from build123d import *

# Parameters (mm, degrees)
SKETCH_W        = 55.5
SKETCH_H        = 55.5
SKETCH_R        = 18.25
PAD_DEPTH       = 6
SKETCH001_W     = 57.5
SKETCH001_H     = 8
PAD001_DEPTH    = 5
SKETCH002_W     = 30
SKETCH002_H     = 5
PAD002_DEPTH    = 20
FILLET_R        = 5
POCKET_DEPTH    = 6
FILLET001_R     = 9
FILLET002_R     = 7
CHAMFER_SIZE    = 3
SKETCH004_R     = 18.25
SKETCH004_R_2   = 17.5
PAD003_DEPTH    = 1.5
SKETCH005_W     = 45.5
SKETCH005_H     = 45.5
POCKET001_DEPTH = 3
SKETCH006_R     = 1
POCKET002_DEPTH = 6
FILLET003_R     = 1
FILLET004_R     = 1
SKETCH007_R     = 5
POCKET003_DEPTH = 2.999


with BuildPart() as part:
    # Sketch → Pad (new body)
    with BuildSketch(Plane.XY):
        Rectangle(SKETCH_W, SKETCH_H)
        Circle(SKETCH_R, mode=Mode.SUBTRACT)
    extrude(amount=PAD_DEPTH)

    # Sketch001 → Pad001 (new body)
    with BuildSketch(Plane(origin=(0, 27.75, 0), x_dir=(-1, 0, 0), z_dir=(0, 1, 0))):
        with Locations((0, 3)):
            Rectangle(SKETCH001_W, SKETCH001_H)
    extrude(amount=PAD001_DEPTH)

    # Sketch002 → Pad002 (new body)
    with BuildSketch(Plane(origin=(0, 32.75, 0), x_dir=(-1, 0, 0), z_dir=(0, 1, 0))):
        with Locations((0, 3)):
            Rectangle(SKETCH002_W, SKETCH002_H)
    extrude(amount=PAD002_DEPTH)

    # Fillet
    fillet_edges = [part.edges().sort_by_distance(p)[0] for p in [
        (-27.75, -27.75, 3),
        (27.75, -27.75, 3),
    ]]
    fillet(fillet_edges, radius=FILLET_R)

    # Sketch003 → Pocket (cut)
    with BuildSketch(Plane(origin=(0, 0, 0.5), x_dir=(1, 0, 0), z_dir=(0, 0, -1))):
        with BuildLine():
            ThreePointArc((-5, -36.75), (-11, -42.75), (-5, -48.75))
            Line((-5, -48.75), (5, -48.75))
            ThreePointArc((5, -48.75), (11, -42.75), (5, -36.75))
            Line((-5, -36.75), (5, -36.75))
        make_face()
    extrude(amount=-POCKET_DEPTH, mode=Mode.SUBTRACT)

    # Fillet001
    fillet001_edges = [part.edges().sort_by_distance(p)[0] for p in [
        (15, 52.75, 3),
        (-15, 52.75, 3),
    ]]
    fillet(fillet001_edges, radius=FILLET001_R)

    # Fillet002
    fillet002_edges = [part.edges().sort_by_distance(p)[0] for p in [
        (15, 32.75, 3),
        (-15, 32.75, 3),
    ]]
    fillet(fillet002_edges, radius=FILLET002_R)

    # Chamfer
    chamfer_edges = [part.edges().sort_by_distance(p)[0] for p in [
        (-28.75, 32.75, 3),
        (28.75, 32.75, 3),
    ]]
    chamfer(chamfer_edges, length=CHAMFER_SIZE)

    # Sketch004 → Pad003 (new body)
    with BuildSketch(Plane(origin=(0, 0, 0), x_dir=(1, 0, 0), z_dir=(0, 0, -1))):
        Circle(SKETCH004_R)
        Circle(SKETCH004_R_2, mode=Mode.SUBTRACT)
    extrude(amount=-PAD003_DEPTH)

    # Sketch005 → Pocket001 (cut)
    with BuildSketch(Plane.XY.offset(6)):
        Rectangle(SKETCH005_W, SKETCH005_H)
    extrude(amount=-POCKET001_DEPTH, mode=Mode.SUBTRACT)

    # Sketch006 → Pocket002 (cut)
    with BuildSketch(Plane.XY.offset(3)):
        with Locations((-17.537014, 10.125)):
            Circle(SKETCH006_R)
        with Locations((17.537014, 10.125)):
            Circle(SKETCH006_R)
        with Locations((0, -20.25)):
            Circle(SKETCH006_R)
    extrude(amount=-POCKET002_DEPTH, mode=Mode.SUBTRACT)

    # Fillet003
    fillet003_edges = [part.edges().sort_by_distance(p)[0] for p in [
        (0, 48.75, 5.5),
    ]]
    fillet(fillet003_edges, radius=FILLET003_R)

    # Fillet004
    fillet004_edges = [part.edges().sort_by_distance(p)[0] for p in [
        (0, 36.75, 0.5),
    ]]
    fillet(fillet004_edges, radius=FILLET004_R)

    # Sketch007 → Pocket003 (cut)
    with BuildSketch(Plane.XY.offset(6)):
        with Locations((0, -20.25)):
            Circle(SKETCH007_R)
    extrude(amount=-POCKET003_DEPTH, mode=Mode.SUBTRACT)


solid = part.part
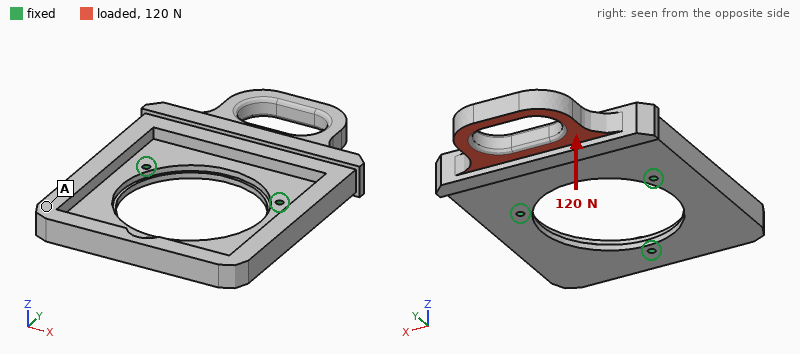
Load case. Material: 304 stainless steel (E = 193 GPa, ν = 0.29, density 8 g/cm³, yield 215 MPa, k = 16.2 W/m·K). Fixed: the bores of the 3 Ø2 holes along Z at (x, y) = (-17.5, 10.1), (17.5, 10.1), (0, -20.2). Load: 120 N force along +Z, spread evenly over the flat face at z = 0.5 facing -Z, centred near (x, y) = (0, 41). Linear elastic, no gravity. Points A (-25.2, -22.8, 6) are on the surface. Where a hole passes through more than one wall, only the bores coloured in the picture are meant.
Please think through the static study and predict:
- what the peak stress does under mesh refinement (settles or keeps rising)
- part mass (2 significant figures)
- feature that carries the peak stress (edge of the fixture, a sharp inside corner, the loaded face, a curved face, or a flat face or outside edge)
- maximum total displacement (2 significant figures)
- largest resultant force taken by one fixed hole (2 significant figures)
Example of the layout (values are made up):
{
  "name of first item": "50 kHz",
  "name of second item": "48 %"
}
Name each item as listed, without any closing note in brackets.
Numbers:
{
  "what the peak stress does under mesh refinement": "keeps rising",
  "part mass": "100 g",
  "feature that carries the peak stress": "edge of the fixture",
  "maximum total displacement": "62 µm",
  "largest resultant force taken by one fixed hole": "98 N"
}
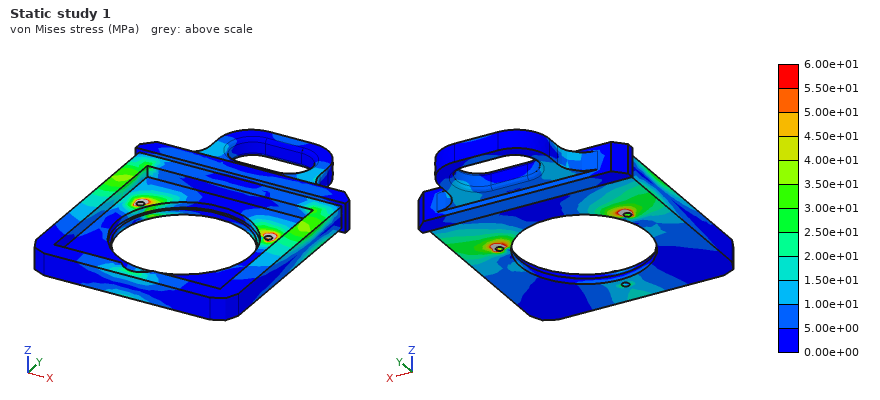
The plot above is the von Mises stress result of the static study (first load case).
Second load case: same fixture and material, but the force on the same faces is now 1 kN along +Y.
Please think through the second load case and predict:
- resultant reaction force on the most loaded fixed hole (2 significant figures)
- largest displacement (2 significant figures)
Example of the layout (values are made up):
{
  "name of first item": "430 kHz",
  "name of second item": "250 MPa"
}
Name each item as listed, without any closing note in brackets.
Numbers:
{
  "resultant reaction force on the most loaded fixed hole": "500 N",
  "largest displacement": "36 µm"
}
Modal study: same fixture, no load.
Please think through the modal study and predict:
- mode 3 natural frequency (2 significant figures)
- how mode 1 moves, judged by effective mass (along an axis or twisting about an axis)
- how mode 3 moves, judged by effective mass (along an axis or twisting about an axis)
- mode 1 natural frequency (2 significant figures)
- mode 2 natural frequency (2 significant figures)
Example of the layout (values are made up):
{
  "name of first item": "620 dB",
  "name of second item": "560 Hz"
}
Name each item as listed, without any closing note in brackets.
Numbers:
{
  "mode 3 natural frequency": "4900 Hz",
  "how mode 1 moves, judged by effective mass": "along Z",
  "how mode 3 moves, judged by effective mass": "along Z",
  "mode 1 natural frequency": "1800 Hz",
  "mode 2 natural frequency": "3300 Hz"
}
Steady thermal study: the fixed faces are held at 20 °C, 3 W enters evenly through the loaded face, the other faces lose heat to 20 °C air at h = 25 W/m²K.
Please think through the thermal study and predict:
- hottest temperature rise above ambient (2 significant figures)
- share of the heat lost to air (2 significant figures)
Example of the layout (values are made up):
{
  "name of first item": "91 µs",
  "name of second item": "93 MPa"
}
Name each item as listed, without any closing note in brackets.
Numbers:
{
  "hottest temperature rise above ambient": "39 K",
  "share of the heat lost to air": "57 %"
}
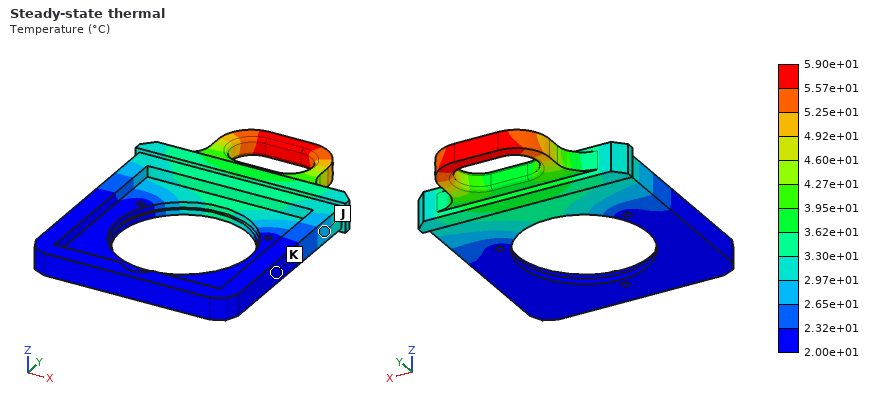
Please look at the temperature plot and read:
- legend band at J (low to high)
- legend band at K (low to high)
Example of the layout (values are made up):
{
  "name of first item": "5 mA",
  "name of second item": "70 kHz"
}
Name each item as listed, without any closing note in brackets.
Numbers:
{
  "legend band at J": "2.65e+01 to 2.97e+01 °C",
  "legend band at K": "2.00e+01 to 2.32e+01 °C"
}
